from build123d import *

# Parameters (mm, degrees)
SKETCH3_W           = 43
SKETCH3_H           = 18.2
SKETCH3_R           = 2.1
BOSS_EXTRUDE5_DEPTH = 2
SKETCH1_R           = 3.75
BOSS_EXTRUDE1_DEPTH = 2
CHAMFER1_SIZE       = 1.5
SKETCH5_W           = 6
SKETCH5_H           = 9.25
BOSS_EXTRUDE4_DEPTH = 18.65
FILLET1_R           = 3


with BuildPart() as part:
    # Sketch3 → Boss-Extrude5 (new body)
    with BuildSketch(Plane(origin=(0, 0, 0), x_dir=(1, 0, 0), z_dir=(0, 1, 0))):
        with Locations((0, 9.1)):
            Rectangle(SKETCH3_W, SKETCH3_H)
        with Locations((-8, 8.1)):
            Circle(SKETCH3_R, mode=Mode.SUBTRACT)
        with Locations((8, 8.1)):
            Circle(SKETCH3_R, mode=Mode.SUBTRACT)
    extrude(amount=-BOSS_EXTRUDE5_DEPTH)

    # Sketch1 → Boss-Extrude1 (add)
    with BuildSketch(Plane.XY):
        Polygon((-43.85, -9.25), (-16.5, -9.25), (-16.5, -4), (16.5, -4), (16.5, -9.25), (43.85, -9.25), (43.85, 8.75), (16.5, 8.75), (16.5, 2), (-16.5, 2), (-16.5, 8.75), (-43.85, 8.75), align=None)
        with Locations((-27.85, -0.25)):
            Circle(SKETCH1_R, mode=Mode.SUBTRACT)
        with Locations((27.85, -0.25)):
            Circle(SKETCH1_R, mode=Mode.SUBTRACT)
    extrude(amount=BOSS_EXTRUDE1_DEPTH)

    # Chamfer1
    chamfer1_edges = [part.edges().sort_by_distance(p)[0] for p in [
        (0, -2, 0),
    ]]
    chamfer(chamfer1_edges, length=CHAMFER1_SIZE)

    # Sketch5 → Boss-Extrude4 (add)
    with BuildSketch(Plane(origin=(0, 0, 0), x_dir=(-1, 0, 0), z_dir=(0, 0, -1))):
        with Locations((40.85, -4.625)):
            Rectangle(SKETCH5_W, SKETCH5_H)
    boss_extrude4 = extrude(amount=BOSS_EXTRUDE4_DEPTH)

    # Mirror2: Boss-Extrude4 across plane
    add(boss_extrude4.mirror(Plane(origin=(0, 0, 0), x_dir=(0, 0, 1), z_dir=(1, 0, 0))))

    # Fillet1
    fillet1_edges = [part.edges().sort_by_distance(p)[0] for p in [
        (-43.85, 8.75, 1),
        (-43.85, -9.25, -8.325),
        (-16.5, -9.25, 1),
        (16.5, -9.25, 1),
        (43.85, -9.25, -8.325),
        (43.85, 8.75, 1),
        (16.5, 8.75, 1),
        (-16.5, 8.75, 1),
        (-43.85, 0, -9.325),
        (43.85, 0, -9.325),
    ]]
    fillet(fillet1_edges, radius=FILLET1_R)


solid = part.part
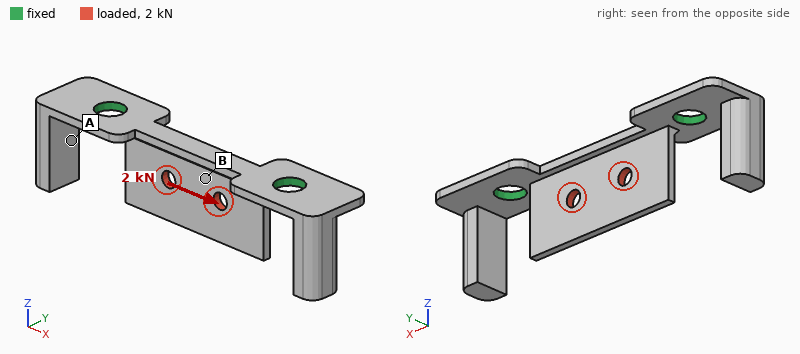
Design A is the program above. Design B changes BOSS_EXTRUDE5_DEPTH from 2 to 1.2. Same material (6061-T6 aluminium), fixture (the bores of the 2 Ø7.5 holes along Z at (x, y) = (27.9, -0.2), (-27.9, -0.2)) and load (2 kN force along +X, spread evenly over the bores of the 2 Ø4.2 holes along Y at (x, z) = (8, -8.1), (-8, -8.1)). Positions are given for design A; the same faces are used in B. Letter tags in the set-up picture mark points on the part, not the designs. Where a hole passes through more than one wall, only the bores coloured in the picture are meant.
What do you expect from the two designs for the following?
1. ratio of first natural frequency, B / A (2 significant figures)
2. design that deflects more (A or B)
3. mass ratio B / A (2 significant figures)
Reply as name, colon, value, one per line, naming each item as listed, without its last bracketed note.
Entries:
ratio of first natural frequency, B / A: 0.99
design that deflects more: B
mass ratio B / A: 0.89
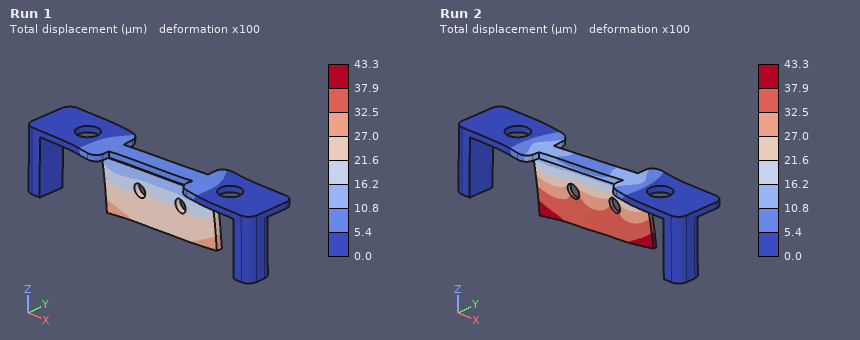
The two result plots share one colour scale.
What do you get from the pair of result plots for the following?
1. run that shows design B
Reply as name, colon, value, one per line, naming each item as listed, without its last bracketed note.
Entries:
run that shows design B: Run 2
